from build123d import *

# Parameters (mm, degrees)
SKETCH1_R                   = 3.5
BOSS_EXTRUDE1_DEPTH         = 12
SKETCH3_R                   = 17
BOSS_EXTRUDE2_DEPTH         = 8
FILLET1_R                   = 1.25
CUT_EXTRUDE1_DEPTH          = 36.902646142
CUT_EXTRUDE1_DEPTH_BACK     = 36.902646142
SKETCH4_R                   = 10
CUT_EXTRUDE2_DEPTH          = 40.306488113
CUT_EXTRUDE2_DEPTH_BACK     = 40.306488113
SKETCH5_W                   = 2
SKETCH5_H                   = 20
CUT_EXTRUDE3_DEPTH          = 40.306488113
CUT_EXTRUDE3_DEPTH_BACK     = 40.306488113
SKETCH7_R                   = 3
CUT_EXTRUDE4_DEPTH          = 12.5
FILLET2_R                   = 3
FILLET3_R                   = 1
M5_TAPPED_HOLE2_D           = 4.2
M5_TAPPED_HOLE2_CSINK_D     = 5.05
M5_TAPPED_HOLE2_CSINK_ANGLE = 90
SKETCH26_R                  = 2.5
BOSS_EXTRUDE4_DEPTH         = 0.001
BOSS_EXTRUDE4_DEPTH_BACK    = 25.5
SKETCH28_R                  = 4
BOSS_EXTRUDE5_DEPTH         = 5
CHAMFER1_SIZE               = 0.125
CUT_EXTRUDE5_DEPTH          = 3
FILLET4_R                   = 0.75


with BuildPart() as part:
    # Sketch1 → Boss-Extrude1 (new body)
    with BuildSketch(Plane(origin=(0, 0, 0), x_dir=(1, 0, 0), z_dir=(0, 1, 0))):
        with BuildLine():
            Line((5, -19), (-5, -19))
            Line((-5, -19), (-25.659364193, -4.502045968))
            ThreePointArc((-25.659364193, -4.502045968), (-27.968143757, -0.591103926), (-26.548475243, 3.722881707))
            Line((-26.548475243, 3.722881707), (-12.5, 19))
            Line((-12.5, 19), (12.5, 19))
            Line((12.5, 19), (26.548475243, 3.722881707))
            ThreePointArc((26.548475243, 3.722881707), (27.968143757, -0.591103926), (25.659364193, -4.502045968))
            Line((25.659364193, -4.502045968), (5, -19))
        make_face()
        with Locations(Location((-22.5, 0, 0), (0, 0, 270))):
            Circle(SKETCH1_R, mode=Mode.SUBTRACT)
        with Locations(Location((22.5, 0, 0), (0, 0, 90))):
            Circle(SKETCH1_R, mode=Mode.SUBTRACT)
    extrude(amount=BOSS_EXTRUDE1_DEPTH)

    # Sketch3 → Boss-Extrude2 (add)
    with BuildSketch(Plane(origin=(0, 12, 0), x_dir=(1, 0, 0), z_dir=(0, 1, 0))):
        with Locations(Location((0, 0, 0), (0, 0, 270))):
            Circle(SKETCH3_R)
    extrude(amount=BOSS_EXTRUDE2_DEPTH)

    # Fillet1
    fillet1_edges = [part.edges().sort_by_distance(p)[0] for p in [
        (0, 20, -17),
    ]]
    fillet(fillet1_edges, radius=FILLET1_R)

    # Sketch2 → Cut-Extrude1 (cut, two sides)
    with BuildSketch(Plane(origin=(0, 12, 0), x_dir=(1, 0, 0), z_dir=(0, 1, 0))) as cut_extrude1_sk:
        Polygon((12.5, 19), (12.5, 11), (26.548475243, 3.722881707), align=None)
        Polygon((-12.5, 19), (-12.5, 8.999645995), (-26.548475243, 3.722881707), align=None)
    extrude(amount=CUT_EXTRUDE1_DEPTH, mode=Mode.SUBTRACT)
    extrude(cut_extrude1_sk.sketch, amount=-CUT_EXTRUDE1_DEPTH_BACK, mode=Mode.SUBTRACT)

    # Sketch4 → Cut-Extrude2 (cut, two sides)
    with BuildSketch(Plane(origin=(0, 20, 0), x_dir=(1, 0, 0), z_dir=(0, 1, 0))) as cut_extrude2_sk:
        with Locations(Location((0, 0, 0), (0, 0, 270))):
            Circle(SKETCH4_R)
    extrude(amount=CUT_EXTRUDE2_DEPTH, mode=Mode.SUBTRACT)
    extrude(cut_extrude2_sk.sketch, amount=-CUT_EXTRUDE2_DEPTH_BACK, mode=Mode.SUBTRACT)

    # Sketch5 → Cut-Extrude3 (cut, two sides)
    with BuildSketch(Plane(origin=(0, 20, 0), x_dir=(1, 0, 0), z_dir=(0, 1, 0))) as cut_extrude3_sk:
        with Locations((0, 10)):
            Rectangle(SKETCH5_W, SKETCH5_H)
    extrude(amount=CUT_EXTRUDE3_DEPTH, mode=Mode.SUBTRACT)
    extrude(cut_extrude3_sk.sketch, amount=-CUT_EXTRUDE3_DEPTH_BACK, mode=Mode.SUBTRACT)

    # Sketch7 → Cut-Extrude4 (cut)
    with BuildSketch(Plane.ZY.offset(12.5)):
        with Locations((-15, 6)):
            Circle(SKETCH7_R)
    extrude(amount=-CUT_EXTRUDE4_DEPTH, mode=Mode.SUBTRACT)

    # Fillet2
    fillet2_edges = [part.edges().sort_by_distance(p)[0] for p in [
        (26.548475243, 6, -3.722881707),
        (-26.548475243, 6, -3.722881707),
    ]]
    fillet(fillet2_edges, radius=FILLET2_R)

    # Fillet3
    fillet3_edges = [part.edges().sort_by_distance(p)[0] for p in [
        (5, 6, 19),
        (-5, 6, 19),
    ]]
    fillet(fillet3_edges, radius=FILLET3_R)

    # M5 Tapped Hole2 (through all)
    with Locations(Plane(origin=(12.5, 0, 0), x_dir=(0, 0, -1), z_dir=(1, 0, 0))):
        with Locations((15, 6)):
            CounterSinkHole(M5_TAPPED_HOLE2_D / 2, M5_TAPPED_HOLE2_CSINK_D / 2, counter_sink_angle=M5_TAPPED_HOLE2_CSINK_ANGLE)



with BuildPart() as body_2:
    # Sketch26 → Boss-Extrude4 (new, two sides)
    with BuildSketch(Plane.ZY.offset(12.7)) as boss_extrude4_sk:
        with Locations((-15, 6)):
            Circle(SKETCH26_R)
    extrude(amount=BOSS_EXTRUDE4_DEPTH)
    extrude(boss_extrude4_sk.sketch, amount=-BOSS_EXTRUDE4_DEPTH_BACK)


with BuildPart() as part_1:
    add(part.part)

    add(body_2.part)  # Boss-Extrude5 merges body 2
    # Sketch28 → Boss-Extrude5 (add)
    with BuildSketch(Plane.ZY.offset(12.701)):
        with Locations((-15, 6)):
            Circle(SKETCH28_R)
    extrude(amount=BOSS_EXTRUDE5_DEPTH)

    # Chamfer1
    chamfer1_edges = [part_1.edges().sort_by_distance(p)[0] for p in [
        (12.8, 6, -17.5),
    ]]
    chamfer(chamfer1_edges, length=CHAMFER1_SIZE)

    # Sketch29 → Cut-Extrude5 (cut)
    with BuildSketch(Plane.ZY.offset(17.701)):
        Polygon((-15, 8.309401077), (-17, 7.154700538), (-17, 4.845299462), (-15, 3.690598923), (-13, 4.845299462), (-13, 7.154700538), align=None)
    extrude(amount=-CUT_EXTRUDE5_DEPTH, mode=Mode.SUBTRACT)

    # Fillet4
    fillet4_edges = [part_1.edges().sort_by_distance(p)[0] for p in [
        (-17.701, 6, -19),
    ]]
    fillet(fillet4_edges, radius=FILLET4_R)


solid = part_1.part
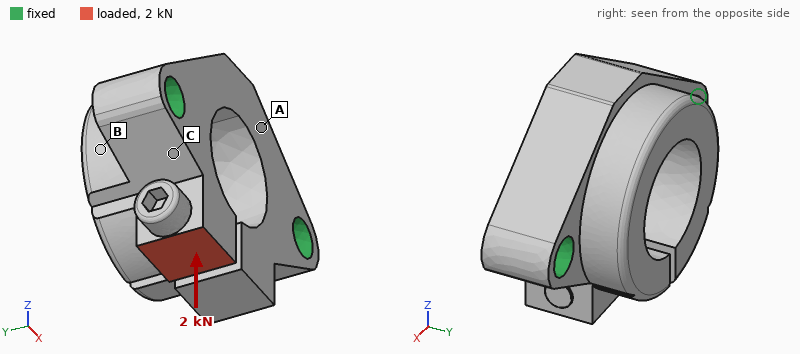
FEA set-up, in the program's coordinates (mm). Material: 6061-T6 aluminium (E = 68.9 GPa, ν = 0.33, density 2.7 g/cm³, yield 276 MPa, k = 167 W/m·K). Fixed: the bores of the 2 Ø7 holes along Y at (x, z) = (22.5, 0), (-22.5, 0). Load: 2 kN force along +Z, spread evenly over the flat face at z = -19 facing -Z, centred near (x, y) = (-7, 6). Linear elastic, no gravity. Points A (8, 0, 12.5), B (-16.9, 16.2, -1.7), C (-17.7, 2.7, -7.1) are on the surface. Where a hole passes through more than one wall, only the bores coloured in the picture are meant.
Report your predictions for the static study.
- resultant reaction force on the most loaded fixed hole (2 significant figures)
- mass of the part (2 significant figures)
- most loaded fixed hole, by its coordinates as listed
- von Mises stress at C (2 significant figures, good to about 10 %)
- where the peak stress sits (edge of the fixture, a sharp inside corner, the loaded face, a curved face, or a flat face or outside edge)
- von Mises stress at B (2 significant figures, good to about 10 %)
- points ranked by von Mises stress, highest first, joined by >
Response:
1.8 kN
44 g
(-22.5, 0)
50 MPa
a curved face
29 MPa
C > B > A
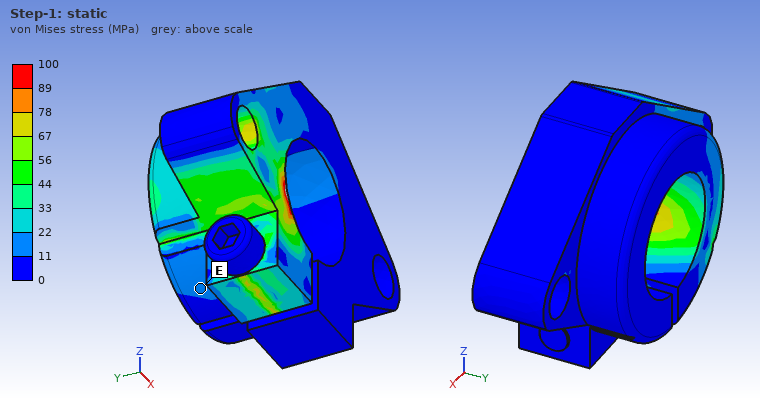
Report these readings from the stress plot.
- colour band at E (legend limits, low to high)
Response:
11 to 22 MPa
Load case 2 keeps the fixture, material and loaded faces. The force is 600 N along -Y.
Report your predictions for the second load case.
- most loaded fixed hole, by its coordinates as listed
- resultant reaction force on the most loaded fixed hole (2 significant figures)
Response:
(-22.5, 0)
610 N
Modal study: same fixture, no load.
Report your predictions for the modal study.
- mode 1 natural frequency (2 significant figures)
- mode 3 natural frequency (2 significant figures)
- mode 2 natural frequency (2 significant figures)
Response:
5600 Hz
11 kHz
6000 Hz
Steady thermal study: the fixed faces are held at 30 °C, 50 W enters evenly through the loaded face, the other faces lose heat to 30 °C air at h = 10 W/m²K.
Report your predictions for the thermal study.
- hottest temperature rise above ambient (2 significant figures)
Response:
68 K
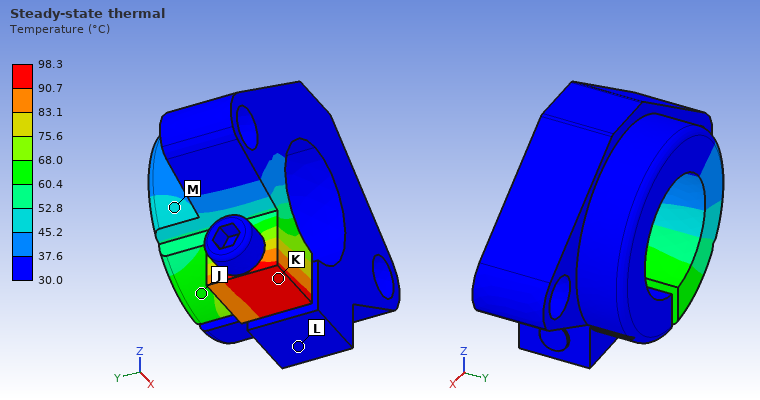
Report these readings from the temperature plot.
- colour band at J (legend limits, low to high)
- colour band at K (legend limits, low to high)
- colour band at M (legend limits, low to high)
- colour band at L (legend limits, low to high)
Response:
60.4 to 68.0 °C
90.7 to 98.3 °C
45.2 to 52.8 °C
30.0 to 37.6 °C
